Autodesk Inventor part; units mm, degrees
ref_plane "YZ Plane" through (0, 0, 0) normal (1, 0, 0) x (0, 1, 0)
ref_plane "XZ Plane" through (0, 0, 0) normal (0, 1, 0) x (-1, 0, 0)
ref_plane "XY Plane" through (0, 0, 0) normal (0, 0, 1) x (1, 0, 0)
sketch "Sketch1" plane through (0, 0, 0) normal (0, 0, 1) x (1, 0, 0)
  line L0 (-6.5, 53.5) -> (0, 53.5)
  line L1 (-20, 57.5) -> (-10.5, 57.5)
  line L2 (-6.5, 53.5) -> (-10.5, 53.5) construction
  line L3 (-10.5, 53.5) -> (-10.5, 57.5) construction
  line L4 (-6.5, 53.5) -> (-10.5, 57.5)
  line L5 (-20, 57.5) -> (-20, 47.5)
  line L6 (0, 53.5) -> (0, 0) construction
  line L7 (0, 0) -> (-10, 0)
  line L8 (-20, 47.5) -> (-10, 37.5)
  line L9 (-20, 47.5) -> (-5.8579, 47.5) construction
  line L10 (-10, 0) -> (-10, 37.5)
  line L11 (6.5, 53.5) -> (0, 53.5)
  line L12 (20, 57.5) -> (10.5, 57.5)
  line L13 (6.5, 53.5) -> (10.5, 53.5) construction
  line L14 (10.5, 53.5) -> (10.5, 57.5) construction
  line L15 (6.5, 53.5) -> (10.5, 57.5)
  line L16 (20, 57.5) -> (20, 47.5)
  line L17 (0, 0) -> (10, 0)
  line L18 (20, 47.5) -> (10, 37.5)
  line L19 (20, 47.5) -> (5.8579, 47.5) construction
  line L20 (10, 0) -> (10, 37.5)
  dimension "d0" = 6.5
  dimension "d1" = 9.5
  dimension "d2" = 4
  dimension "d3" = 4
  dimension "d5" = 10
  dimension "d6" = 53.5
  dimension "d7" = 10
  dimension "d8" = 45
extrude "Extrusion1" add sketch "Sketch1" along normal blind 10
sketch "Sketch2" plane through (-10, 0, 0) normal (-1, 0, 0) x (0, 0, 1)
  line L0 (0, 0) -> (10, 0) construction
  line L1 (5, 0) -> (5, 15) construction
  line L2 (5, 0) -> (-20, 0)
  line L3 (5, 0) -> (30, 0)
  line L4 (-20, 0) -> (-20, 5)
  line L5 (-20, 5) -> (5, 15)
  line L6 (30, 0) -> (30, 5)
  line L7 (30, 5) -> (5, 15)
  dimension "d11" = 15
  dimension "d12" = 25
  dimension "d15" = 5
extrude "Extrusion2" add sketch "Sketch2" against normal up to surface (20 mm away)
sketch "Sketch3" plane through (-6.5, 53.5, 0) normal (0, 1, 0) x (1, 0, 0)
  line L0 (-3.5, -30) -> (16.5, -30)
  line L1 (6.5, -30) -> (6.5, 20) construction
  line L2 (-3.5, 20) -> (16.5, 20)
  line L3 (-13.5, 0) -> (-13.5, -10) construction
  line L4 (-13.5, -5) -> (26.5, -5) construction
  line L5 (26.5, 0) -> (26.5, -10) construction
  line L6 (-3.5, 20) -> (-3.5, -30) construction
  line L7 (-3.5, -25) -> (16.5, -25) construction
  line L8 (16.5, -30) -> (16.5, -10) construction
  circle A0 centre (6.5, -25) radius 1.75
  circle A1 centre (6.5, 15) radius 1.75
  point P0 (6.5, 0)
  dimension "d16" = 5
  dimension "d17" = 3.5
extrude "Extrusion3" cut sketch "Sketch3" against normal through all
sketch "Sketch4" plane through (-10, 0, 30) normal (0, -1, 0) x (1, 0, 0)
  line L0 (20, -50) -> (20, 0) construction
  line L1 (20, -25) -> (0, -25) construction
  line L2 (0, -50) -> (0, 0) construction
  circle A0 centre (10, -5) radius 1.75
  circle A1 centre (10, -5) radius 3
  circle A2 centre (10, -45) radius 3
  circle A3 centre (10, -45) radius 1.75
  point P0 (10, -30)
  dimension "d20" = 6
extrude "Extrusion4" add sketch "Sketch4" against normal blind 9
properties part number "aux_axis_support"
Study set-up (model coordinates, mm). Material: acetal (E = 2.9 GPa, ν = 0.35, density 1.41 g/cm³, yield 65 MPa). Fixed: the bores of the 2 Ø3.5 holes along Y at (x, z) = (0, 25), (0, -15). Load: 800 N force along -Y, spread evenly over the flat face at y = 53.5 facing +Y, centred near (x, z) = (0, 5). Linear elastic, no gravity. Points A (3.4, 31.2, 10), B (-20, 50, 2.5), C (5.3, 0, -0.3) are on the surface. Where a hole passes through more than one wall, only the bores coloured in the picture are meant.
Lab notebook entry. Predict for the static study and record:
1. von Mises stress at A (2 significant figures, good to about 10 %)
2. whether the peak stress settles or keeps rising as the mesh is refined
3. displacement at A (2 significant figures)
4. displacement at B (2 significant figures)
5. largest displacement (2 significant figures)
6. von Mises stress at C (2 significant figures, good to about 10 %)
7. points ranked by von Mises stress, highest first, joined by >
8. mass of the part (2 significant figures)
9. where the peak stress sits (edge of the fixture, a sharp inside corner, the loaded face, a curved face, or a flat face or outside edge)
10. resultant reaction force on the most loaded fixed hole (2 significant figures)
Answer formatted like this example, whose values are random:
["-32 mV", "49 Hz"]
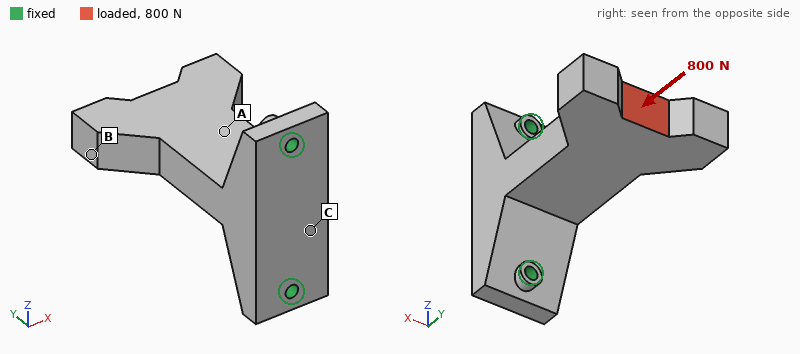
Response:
["3.9 MPa", "keeps rising", "0.11 mm", "0.11 mm", "0.14 mm", "5.4 MPa", "C > A > B", "30 g", "edge of the fixture", "450 N"]
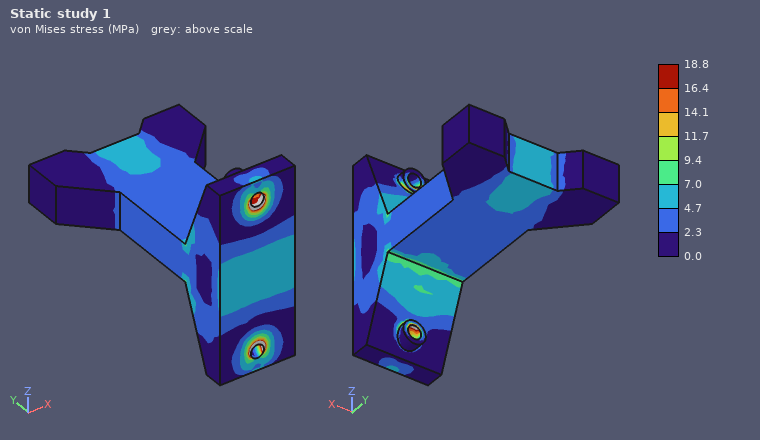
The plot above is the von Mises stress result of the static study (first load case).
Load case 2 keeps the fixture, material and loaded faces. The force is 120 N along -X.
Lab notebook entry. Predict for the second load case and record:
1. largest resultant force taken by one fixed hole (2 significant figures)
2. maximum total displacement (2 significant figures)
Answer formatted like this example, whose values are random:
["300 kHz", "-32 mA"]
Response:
["60 N", "0.97 mm"]
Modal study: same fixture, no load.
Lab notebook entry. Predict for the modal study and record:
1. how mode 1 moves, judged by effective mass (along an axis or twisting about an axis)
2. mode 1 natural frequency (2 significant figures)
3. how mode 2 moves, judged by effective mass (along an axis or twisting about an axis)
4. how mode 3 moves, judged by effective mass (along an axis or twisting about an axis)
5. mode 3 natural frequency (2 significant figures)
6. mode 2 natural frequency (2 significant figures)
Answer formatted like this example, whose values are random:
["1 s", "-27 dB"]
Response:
["along X", "650 Hz", "along Z", "twisting about Y", "1800 Hz", "760 Hz"]
